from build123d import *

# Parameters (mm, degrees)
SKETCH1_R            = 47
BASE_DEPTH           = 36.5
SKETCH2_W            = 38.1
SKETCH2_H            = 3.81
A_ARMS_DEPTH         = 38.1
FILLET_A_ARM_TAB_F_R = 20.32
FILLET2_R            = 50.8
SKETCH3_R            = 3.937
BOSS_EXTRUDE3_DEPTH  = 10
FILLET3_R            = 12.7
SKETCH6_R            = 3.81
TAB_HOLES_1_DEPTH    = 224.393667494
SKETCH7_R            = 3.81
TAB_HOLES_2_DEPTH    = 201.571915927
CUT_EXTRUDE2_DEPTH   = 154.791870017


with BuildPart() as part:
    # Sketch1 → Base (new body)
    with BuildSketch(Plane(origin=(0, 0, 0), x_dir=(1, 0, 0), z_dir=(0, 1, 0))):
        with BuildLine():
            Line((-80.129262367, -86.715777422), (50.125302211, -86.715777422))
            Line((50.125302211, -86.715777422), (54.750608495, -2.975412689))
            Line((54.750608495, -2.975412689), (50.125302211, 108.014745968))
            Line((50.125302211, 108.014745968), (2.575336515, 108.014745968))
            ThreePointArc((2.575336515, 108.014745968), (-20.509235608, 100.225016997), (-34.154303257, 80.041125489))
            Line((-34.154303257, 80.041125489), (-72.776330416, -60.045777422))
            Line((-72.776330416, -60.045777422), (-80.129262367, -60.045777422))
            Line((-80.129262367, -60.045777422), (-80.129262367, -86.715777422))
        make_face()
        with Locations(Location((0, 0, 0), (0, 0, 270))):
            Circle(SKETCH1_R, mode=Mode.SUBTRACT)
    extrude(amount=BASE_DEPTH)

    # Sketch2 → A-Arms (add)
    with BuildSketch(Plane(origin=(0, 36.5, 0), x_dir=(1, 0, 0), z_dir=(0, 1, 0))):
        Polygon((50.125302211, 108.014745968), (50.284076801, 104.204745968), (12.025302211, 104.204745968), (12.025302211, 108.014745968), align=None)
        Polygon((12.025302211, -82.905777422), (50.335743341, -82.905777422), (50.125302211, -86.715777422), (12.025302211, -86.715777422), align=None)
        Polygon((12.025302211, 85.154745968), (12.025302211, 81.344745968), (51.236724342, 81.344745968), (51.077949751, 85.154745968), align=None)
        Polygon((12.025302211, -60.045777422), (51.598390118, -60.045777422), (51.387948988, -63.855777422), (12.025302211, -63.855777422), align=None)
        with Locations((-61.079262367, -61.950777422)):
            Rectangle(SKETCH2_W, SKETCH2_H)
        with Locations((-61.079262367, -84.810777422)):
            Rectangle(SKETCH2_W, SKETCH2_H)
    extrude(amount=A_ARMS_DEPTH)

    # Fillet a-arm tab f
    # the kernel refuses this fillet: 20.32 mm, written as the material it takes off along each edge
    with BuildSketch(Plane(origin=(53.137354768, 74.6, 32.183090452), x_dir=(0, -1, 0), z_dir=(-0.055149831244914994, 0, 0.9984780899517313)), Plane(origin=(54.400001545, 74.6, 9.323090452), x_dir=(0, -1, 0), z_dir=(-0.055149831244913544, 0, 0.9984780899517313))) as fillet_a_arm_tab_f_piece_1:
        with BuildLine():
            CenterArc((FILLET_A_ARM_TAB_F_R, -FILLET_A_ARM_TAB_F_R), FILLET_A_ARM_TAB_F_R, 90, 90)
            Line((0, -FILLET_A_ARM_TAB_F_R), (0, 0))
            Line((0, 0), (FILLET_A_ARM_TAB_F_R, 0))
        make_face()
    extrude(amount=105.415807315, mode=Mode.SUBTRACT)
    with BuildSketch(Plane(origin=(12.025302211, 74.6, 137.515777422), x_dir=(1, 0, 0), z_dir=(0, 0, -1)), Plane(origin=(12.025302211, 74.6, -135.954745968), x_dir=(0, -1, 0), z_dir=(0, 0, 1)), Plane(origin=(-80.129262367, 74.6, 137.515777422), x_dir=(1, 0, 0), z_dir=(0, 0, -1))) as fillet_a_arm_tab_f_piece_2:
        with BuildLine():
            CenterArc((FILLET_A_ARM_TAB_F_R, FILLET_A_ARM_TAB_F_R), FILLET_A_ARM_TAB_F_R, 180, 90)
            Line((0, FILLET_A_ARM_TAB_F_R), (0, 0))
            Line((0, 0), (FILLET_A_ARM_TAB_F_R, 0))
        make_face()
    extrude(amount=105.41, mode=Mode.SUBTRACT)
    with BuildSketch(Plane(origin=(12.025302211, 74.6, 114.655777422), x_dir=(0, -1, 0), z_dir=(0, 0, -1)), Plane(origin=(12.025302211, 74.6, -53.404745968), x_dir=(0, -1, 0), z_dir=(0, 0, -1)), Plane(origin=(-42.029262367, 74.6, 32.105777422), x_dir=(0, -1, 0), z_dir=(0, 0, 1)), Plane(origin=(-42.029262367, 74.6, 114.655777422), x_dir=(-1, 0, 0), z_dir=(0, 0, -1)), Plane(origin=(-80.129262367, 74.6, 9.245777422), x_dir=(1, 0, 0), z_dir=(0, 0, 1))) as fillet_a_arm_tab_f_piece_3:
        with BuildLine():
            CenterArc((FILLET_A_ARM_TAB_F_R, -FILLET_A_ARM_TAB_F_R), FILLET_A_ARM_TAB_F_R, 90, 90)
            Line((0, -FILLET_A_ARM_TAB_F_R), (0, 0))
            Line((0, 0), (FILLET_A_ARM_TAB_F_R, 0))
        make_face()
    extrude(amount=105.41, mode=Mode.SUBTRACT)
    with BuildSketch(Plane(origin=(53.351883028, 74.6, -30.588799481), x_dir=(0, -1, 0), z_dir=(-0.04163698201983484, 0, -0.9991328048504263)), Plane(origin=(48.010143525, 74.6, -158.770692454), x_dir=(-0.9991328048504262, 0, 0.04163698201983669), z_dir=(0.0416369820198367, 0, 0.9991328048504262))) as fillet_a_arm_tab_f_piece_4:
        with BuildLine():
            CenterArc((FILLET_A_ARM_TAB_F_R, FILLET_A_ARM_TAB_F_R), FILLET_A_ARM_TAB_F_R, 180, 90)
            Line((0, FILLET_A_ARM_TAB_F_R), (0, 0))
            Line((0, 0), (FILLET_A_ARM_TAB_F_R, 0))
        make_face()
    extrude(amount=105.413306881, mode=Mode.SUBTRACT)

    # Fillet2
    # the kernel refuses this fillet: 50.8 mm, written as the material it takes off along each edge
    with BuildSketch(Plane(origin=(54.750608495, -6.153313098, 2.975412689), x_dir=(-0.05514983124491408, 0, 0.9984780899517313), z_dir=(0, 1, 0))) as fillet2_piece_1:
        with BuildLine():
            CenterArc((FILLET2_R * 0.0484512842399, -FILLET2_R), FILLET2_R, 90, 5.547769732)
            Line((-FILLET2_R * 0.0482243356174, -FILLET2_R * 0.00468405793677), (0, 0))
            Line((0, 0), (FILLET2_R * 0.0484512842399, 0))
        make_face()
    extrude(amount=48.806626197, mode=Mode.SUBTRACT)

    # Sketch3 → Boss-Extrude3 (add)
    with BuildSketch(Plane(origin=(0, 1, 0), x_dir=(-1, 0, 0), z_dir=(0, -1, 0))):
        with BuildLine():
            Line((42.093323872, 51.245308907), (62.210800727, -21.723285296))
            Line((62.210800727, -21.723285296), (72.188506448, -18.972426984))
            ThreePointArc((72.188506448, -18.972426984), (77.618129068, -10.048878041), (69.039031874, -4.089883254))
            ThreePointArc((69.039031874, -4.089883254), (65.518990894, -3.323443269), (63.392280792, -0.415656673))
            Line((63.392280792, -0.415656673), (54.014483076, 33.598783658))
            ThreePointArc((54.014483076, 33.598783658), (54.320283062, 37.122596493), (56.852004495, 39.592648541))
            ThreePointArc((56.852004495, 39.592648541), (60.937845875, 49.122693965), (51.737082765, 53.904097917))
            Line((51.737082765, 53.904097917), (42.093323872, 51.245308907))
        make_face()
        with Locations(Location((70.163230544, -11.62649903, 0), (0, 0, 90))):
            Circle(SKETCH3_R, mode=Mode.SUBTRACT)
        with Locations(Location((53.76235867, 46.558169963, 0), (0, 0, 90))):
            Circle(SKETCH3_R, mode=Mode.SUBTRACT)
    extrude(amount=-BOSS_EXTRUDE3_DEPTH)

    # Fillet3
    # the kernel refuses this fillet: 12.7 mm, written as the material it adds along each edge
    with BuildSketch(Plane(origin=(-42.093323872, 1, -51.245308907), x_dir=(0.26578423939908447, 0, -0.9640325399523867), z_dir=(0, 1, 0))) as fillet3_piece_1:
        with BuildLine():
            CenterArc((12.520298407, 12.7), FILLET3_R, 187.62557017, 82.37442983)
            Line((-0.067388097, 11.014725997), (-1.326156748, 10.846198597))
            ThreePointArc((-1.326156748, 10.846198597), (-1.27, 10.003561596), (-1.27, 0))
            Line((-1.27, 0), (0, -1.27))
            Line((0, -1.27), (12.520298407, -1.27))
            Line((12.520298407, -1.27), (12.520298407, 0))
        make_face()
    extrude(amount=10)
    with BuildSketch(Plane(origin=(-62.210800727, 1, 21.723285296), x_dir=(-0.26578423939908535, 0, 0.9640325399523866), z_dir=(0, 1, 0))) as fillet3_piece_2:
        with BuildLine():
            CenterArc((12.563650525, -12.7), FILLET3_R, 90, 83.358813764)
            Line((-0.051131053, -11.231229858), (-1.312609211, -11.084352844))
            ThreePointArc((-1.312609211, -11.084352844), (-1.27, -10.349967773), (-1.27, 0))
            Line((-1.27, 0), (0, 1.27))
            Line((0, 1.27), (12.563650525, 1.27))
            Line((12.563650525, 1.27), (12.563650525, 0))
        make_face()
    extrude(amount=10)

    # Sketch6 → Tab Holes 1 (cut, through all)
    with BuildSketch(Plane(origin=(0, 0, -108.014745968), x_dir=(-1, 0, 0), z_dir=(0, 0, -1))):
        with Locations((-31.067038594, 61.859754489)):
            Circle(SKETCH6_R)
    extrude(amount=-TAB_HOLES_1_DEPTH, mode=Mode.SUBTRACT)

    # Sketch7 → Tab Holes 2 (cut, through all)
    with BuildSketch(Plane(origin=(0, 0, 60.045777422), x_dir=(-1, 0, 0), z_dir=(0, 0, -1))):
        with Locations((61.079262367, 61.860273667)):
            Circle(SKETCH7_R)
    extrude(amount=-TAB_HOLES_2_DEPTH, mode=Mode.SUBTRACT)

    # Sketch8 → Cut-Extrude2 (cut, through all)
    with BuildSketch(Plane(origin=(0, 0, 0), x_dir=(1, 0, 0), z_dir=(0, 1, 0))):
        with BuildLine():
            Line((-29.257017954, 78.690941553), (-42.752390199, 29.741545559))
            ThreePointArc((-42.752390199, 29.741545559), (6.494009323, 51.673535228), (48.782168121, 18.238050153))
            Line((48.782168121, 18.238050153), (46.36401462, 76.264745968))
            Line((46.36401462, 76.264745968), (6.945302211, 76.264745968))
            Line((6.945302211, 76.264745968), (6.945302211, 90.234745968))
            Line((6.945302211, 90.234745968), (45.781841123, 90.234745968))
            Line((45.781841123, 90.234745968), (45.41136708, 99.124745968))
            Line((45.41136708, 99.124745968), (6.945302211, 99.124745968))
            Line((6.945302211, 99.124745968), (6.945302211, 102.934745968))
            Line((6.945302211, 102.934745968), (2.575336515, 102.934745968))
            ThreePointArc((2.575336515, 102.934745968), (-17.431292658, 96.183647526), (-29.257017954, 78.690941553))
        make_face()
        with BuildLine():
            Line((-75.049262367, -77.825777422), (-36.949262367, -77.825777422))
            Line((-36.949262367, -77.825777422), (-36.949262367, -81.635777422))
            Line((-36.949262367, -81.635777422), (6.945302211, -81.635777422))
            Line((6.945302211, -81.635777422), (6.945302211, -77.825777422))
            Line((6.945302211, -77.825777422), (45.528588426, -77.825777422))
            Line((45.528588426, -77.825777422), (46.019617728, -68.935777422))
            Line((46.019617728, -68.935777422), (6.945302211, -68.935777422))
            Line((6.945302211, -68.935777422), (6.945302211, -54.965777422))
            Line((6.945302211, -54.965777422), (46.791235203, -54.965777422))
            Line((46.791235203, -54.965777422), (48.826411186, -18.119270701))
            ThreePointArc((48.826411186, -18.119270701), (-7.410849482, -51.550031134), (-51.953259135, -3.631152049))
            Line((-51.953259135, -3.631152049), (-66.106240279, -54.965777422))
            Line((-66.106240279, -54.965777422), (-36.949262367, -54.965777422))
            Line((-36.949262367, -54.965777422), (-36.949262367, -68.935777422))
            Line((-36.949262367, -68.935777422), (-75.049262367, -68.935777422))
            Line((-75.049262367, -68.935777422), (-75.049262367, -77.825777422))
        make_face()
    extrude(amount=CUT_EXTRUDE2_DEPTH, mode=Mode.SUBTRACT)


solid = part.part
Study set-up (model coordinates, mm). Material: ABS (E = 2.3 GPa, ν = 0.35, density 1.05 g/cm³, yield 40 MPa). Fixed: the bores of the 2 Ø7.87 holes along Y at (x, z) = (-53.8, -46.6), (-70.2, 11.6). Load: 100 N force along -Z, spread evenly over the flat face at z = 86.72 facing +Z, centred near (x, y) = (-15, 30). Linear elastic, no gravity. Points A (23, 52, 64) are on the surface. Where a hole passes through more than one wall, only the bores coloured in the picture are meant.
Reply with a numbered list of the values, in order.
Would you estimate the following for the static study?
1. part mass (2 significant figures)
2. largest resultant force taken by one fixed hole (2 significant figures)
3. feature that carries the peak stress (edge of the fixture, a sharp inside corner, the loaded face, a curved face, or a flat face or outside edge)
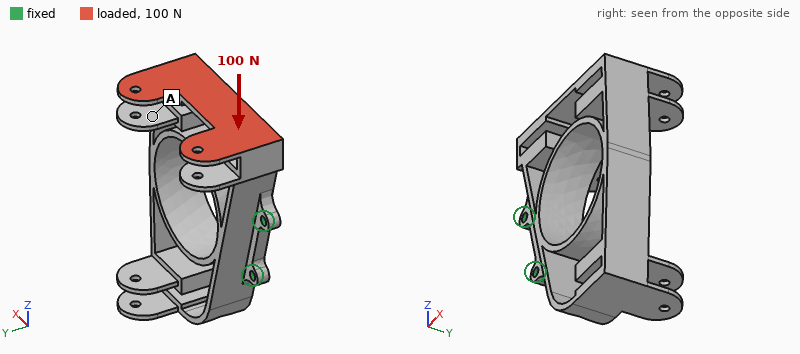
1. 280 g
2. 97 N
3. a flat face or outside edge
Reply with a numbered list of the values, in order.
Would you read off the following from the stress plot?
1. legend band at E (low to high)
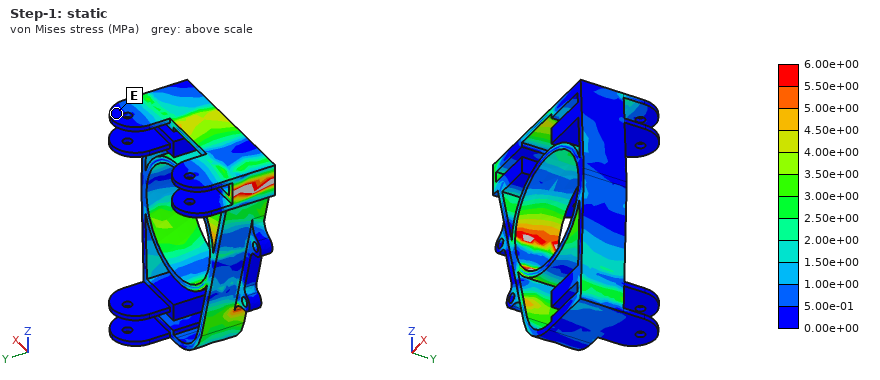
1. 0.00e+00 to 5.00e-01 MPa
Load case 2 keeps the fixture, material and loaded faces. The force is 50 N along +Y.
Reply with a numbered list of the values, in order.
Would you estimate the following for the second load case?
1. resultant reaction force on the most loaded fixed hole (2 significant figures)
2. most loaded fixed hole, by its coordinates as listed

1. 90 N
2. (-70.2, 11.6)
